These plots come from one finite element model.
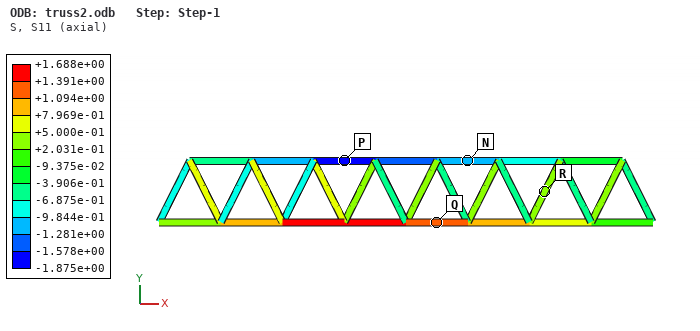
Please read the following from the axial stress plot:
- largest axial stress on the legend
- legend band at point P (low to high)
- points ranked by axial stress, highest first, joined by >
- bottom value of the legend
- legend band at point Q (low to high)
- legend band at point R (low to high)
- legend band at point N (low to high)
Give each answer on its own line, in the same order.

+1.688e+00
-1.875e+00 to -1.578e+00
Q > R > N > P
-1.875e+00
+1.094e+00 to +1.391e+00
+2.031e-01 to +5.000e-01
-1.281e+00 to -9.844e-01
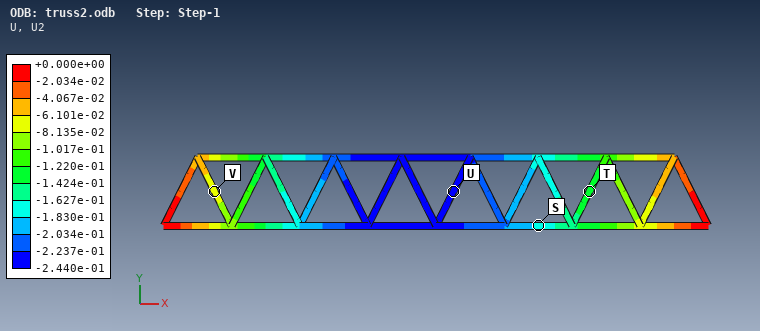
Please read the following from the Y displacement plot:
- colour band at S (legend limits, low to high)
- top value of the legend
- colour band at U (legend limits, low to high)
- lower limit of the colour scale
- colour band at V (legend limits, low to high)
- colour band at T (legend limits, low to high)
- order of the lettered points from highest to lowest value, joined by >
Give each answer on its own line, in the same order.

-1.830e-01 to -1.627e-01
+0.000e+00
-2.440e-01 to -2.237e-01
-2.440e-01
-8.135e-02 to -6.101e-02
-1.424e-01 to -1.220e-01
V > T > S > U
